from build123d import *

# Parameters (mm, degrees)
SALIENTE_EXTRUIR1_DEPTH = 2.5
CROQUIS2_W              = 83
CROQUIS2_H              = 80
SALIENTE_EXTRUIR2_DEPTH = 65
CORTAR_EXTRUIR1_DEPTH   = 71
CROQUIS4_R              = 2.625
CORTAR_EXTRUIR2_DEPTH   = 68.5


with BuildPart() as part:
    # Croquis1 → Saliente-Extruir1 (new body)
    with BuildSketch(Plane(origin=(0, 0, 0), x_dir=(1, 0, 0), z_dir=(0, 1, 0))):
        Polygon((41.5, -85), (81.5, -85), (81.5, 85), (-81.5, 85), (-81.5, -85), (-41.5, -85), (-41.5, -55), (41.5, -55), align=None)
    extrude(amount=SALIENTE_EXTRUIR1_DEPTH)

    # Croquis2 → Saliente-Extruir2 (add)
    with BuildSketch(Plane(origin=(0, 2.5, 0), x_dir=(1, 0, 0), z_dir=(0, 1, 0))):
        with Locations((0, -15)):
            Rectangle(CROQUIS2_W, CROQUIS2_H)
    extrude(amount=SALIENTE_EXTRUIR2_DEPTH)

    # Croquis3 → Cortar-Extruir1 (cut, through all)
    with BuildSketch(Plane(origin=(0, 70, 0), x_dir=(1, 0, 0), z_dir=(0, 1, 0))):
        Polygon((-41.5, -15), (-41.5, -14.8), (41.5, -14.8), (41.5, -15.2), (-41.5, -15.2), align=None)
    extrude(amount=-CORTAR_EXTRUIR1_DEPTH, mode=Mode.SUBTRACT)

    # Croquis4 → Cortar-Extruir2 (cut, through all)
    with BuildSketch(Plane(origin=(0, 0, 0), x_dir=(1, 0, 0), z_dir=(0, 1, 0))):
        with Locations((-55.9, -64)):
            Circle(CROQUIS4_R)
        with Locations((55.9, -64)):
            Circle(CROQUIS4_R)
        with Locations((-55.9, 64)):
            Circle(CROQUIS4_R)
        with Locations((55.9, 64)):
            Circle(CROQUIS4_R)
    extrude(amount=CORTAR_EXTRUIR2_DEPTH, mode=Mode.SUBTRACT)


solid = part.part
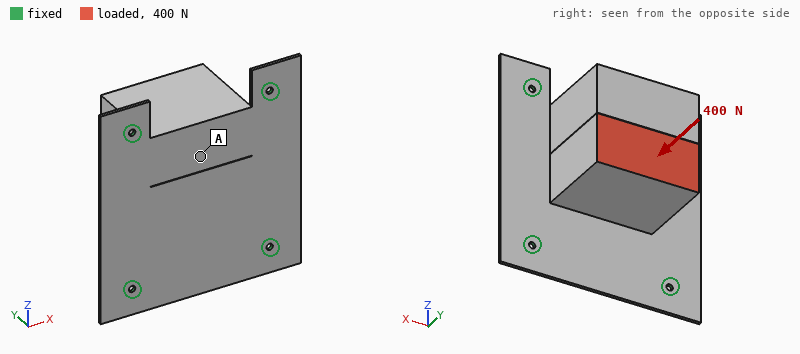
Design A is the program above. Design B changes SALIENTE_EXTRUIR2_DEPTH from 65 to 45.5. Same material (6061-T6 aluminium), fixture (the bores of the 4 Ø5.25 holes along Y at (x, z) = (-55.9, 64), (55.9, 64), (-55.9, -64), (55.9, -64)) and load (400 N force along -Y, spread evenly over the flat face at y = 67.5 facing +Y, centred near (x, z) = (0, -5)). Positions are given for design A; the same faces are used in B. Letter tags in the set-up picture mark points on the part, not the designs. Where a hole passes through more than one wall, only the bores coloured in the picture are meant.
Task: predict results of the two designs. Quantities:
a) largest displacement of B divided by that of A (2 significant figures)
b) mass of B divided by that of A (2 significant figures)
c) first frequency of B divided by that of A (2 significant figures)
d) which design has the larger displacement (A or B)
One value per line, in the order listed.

0.80
0.74
1.4
A
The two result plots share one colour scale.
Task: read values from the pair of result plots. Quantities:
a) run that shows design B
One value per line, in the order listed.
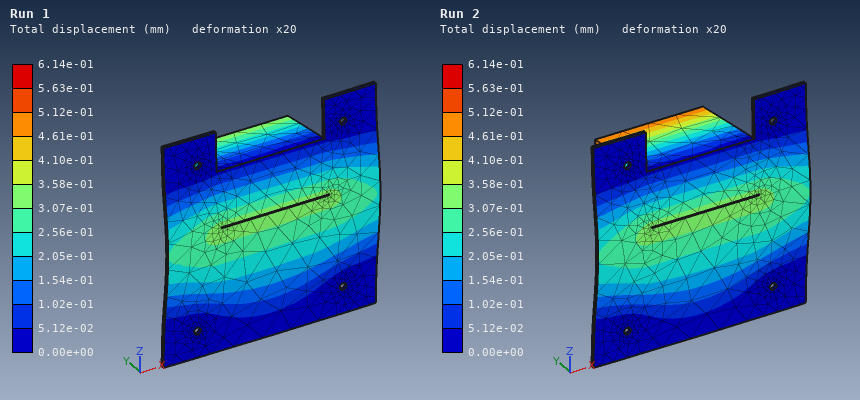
Run 1
